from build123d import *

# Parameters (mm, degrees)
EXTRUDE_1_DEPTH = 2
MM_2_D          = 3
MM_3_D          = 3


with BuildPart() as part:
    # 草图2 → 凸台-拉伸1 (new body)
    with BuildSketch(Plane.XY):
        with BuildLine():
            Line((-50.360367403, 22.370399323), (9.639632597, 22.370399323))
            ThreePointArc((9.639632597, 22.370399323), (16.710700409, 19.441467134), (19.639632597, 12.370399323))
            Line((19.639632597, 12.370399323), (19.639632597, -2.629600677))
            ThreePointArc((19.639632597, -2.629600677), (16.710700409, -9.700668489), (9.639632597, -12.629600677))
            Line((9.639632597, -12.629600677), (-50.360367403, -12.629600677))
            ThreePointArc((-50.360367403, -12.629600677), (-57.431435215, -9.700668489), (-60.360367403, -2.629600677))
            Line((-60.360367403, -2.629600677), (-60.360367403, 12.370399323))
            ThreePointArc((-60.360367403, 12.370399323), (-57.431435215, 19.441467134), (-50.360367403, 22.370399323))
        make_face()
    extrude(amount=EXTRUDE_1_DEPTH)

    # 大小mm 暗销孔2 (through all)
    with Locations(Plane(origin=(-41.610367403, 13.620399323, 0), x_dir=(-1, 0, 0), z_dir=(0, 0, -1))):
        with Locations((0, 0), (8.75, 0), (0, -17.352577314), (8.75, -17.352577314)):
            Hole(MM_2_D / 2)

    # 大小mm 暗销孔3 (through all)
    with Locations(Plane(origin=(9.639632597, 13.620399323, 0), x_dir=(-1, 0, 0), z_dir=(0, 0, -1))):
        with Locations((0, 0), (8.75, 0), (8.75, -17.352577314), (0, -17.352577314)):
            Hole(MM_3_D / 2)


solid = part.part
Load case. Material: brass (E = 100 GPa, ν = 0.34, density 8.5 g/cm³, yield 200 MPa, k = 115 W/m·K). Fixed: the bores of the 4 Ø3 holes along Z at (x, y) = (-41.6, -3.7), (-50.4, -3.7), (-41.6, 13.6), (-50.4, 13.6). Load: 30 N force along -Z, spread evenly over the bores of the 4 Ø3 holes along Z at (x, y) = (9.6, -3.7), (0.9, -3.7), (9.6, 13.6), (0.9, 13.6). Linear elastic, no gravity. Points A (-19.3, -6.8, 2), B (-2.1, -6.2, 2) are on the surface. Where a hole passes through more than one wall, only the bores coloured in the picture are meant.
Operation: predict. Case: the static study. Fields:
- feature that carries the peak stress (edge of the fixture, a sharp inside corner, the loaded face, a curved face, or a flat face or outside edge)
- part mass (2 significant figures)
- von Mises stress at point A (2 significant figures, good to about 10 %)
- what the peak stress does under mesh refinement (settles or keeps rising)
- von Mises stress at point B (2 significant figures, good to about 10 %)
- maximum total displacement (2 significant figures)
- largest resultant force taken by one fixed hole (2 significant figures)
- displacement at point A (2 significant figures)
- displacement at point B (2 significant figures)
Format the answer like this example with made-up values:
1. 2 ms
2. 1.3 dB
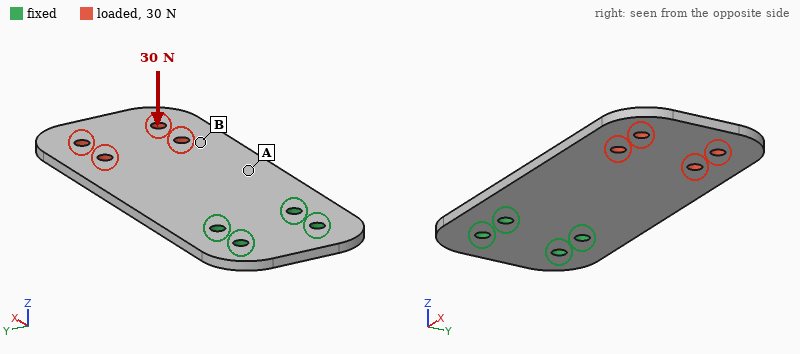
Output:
1. edge of the fixture
2. 45 g
3. 31 MPa
4. keeps rising
5. 11 MPa
6. 0.62 mm
7. 40 N
8. 0.12 mm
9. 0.32 mm
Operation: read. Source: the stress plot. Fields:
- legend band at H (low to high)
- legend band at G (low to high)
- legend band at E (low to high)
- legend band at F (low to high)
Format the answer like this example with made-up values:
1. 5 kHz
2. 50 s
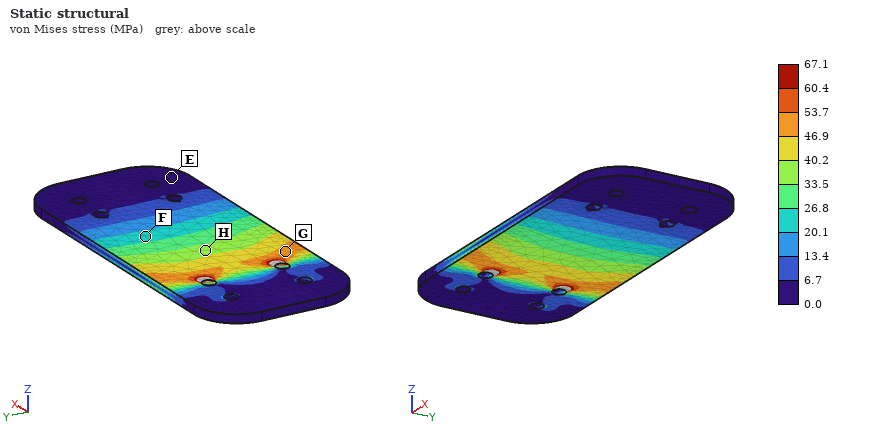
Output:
1. 33.5 to 40.2 MPa
2. 46.9 to 53.7 MPa
3. 0.0 to 6.7 MPa
4. 20.1 to 26.8 MPa
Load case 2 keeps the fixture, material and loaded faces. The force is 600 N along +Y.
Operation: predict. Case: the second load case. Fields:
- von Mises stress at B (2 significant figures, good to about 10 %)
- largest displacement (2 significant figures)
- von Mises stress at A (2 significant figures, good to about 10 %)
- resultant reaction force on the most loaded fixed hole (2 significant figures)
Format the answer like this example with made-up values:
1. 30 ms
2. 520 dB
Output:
1. 13 MPa
2. 69 µm
3. 27 MPa
4. 1.1 kN
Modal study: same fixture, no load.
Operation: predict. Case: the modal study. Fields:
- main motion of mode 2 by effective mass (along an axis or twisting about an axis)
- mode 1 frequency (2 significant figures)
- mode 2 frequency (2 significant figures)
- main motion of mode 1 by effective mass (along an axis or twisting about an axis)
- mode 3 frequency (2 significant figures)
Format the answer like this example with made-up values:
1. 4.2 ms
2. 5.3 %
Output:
1. twisting about X
2. 320 Hz
3. 1200 Hz
4. along Z
5. 1900 Hz
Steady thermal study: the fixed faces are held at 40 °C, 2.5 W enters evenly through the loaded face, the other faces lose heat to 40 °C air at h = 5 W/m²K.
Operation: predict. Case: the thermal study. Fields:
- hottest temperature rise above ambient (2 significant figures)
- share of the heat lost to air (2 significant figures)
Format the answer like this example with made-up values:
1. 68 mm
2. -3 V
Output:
1. 15 K
2. 7.7 %
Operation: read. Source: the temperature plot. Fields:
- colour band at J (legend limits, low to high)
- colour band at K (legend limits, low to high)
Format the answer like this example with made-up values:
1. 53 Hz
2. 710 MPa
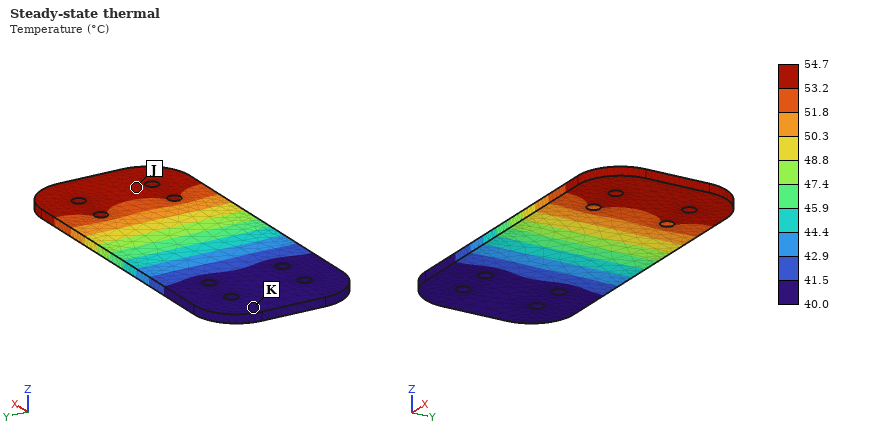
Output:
1. 53.2 to 54.7 °C
2. 40.0 to 41.5 °C
